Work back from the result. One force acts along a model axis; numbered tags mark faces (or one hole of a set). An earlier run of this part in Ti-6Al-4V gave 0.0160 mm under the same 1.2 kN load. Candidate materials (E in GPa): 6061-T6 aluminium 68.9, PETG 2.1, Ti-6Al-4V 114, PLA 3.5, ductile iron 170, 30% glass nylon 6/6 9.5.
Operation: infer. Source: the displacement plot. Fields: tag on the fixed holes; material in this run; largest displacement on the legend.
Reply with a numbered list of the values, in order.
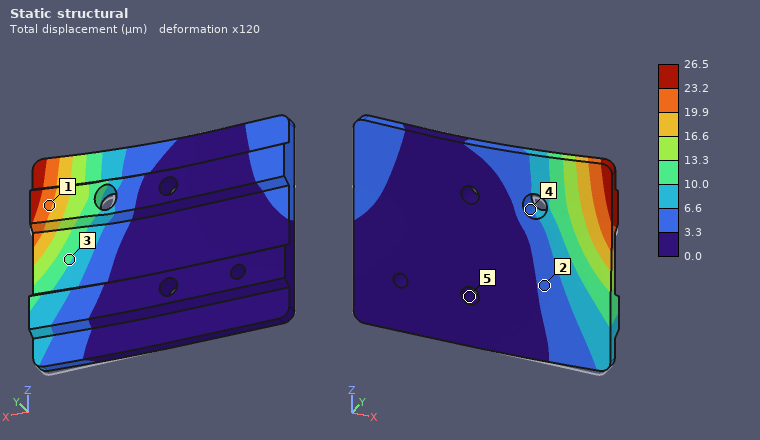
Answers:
1. 5
2. 6061-T6 aluminium
3. 26.5 µm
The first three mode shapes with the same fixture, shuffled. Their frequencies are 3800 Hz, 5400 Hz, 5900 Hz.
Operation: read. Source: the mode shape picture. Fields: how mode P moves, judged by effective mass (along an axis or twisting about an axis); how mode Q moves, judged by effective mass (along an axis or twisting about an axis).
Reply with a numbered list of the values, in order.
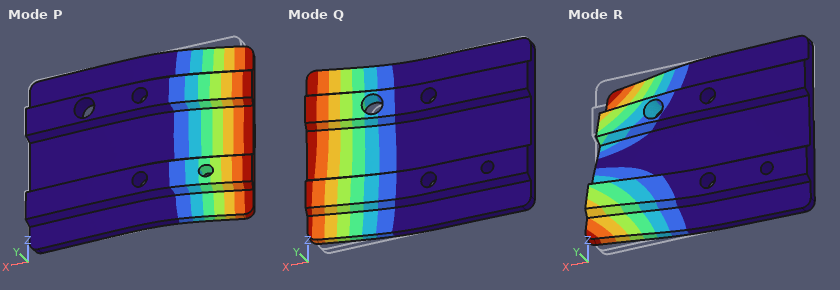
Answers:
1. along Y
2. along Y
